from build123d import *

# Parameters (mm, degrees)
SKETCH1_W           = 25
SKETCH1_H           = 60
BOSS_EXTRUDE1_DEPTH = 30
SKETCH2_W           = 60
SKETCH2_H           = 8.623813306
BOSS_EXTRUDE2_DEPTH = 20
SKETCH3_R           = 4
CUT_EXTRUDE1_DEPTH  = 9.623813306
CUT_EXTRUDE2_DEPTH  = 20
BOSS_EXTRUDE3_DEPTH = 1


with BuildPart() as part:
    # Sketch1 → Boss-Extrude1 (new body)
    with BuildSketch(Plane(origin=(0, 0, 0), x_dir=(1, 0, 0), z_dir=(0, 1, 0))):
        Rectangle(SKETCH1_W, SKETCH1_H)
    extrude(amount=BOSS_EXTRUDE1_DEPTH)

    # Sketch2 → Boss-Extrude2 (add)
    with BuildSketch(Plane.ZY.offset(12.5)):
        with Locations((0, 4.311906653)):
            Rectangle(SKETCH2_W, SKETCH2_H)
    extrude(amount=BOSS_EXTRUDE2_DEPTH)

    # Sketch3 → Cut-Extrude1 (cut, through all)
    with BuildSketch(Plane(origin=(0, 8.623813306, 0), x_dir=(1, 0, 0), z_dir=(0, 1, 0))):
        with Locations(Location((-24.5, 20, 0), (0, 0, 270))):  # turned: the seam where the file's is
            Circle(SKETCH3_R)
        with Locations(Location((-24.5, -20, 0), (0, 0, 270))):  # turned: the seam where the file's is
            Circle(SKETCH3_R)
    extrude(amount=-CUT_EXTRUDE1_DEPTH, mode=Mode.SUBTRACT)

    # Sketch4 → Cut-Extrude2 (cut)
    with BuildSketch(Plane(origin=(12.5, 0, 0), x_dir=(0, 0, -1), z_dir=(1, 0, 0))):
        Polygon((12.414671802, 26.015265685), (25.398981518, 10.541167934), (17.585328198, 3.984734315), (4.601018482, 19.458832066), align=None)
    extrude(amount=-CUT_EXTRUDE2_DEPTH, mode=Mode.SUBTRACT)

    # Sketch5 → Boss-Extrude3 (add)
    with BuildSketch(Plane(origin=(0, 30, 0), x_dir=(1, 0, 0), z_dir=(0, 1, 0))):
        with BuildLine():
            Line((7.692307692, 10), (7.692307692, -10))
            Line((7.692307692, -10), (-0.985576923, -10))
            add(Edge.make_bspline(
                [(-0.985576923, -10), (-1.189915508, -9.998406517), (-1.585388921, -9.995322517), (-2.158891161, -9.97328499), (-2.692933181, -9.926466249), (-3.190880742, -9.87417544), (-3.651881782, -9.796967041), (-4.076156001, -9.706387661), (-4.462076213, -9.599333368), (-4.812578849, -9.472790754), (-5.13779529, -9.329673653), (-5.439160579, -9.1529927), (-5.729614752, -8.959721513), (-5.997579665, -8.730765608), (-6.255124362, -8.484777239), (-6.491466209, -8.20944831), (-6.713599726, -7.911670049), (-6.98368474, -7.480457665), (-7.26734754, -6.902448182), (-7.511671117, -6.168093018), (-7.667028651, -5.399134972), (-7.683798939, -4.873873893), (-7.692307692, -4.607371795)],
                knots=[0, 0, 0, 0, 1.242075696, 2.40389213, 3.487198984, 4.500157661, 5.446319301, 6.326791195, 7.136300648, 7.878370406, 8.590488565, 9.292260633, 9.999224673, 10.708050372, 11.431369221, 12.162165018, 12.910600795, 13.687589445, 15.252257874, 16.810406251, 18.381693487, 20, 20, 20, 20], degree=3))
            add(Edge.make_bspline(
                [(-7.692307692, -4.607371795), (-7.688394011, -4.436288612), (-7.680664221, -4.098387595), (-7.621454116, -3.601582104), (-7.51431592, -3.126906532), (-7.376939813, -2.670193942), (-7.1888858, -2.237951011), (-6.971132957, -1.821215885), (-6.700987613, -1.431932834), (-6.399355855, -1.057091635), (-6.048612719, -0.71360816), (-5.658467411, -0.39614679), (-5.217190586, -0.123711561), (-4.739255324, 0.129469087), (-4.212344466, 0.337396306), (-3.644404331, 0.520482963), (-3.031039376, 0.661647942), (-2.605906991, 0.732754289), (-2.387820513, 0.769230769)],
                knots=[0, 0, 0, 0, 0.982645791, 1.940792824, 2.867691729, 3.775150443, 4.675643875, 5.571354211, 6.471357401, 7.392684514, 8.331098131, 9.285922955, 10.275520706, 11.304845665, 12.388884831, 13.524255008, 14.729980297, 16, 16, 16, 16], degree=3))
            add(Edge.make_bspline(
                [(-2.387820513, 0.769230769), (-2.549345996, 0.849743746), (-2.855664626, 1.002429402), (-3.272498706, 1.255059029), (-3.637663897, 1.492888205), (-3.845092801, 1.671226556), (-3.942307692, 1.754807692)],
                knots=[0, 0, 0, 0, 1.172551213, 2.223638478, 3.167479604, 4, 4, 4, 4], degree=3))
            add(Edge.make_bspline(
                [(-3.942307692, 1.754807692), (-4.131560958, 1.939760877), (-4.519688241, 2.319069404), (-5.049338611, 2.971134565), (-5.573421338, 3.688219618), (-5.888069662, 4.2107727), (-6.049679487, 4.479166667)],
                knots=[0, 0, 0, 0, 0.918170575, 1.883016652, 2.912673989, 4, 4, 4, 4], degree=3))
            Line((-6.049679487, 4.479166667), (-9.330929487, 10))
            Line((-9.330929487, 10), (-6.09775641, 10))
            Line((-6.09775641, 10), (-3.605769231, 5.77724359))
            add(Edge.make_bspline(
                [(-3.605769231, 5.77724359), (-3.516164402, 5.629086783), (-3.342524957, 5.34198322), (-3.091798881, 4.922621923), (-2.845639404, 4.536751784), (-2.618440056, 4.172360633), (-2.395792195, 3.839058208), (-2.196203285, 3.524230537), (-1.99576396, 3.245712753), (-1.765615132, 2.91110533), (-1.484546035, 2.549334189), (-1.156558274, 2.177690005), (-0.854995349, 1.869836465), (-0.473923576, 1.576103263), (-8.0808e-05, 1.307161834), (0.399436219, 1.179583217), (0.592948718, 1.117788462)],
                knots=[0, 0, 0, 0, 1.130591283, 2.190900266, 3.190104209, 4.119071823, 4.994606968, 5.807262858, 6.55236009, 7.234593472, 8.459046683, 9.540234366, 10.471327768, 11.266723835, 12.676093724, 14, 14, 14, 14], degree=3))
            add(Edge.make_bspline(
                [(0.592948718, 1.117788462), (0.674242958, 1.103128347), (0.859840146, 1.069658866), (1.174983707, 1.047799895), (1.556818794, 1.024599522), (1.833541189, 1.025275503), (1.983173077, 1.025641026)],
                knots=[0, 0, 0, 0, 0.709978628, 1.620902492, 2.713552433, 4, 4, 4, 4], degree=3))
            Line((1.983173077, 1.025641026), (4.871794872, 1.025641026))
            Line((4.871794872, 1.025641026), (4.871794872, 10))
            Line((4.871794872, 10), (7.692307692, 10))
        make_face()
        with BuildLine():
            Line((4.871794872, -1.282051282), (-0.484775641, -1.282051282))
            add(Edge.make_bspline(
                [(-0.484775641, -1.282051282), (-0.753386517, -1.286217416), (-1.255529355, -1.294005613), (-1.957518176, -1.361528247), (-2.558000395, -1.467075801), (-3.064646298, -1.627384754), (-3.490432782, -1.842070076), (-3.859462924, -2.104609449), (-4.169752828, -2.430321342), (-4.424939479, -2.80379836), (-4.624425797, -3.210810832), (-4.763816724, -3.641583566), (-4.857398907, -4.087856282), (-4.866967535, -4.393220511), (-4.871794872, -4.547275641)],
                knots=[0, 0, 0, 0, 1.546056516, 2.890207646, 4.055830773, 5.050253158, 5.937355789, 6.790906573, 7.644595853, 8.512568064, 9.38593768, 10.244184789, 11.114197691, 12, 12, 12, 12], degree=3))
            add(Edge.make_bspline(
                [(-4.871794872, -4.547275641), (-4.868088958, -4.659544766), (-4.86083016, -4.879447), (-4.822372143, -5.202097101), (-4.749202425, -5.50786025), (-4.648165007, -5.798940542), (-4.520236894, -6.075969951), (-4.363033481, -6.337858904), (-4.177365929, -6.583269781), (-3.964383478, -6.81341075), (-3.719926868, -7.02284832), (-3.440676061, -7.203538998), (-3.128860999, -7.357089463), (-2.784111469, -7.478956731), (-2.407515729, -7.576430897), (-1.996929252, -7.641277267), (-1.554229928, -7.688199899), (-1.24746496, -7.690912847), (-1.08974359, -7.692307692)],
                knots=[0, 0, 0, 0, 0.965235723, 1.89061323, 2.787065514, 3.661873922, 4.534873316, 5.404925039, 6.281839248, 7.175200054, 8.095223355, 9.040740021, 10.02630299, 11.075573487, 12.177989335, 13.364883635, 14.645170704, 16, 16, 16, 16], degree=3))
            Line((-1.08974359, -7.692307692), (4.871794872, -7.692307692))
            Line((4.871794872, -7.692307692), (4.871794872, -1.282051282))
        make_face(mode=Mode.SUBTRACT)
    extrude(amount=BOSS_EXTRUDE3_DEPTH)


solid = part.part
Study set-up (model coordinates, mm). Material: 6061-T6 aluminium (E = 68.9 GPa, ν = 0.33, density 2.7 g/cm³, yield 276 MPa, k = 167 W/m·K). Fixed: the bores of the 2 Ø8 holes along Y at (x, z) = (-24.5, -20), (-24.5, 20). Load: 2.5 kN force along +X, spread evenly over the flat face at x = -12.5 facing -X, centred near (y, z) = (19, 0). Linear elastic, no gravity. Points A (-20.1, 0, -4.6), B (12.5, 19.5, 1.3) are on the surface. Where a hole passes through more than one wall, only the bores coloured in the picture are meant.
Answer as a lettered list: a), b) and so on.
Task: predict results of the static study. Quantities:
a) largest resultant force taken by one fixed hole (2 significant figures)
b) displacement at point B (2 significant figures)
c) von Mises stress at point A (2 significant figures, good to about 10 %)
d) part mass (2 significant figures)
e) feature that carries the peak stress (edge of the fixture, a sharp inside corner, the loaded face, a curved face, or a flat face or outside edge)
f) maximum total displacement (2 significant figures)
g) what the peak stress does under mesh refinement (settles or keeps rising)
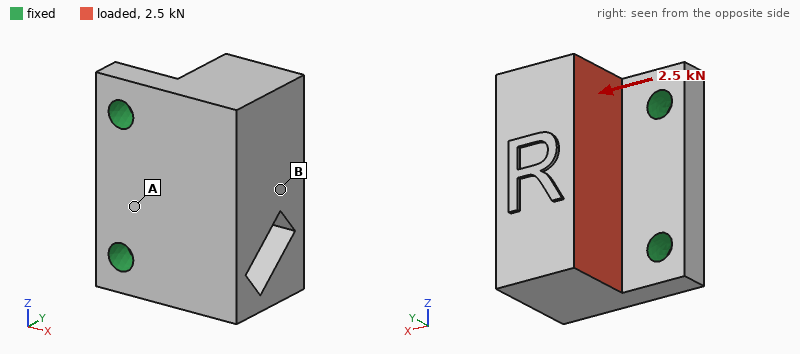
a) 1.3 kN
b) 0.086 mm
c) 24 MPa
d) 140 g
e) edge of the fixture
f) 0.10 mm
g) keeps rising
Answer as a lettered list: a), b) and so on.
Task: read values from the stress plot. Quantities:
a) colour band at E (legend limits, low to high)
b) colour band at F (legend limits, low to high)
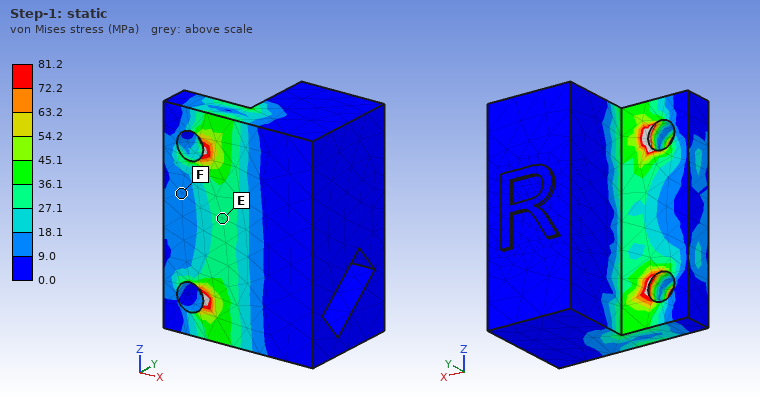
a) 27.1 to 36.1 MPa
b) 9.0 to 18.1 MPa
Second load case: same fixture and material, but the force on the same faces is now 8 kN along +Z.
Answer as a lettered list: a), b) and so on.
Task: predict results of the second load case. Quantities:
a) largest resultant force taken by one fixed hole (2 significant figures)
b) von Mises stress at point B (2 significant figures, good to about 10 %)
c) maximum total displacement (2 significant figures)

a) 5.2 kN
b) 14 MPa
c) 59 µm
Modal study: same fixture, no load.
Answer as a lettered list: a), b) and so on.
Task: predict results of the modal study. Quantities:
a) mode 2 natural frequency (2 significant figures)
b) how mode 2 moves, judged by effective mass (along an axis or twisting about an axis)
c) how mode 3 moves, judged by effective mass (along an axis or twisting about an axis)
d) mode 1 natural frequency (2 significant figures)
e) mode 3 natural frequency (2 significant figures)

a) 6800 Hz
b) along Z
c) along Z
d) 2500 Hz
e) 9800 Hz
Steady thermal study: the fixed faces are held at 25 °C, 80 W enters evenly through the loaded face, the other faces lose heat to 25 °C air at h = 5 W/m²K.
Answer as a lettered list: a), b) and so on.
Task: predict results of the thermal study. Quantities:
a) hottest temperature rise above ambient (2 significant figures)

a) 24 K
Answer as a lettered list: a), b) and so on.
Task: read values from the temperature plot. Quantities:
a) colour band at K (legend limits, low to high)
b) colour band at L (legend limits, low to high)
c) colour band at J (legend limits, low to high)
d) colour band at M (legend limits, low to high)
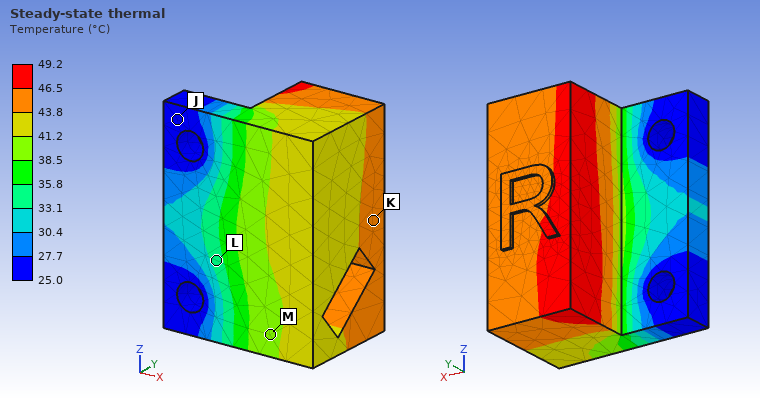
a) 43.8 to 46.5 °C
b) 33.1 to 35.8 °C
c) 25.0 to 27.7 °C
d) 38.5 to 41.2 °C
